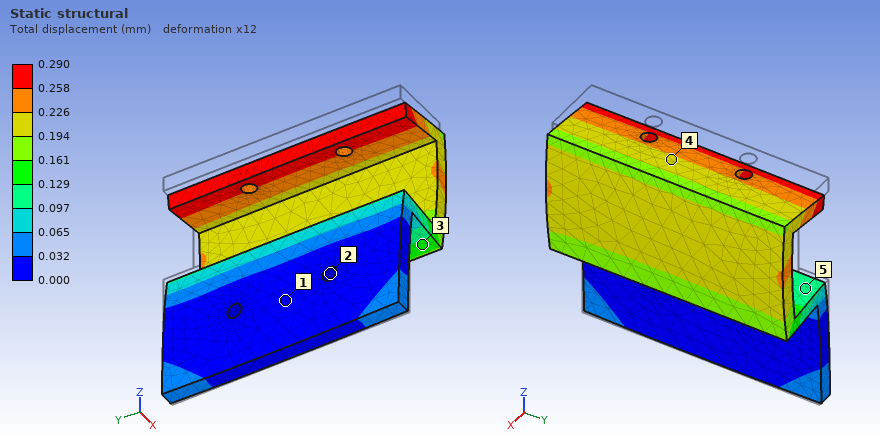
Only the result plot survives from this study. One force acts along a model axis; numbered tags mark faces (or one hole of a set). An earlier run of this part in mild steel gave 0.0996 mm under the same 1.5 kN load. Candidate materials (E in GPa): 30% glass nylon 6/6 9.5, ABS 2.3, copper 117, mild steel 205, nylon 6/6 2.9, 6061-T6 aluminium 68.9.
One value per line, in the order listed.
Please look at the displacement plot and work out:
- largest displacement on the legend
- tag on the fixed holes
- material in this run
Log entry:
0.290 mm
2
6061-T6 aluminium
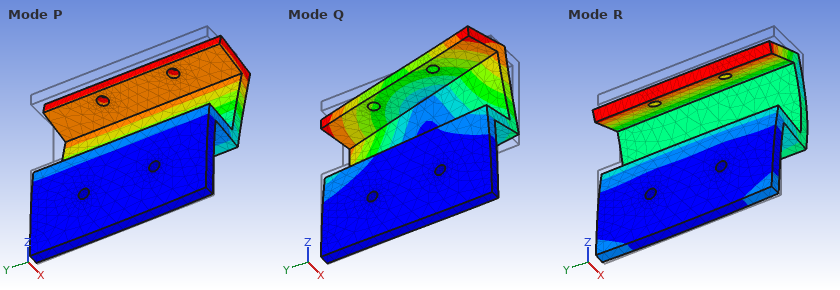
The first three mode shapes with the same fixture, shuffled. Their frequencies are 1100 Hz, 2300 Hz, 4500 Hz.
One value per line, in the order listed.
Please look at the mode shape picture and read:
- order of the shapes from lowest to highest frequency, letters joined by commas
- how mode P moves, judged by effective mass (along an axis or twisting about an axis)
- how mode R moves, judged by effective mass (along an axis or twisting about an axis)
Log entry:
P, Q, R
along X
along Z
